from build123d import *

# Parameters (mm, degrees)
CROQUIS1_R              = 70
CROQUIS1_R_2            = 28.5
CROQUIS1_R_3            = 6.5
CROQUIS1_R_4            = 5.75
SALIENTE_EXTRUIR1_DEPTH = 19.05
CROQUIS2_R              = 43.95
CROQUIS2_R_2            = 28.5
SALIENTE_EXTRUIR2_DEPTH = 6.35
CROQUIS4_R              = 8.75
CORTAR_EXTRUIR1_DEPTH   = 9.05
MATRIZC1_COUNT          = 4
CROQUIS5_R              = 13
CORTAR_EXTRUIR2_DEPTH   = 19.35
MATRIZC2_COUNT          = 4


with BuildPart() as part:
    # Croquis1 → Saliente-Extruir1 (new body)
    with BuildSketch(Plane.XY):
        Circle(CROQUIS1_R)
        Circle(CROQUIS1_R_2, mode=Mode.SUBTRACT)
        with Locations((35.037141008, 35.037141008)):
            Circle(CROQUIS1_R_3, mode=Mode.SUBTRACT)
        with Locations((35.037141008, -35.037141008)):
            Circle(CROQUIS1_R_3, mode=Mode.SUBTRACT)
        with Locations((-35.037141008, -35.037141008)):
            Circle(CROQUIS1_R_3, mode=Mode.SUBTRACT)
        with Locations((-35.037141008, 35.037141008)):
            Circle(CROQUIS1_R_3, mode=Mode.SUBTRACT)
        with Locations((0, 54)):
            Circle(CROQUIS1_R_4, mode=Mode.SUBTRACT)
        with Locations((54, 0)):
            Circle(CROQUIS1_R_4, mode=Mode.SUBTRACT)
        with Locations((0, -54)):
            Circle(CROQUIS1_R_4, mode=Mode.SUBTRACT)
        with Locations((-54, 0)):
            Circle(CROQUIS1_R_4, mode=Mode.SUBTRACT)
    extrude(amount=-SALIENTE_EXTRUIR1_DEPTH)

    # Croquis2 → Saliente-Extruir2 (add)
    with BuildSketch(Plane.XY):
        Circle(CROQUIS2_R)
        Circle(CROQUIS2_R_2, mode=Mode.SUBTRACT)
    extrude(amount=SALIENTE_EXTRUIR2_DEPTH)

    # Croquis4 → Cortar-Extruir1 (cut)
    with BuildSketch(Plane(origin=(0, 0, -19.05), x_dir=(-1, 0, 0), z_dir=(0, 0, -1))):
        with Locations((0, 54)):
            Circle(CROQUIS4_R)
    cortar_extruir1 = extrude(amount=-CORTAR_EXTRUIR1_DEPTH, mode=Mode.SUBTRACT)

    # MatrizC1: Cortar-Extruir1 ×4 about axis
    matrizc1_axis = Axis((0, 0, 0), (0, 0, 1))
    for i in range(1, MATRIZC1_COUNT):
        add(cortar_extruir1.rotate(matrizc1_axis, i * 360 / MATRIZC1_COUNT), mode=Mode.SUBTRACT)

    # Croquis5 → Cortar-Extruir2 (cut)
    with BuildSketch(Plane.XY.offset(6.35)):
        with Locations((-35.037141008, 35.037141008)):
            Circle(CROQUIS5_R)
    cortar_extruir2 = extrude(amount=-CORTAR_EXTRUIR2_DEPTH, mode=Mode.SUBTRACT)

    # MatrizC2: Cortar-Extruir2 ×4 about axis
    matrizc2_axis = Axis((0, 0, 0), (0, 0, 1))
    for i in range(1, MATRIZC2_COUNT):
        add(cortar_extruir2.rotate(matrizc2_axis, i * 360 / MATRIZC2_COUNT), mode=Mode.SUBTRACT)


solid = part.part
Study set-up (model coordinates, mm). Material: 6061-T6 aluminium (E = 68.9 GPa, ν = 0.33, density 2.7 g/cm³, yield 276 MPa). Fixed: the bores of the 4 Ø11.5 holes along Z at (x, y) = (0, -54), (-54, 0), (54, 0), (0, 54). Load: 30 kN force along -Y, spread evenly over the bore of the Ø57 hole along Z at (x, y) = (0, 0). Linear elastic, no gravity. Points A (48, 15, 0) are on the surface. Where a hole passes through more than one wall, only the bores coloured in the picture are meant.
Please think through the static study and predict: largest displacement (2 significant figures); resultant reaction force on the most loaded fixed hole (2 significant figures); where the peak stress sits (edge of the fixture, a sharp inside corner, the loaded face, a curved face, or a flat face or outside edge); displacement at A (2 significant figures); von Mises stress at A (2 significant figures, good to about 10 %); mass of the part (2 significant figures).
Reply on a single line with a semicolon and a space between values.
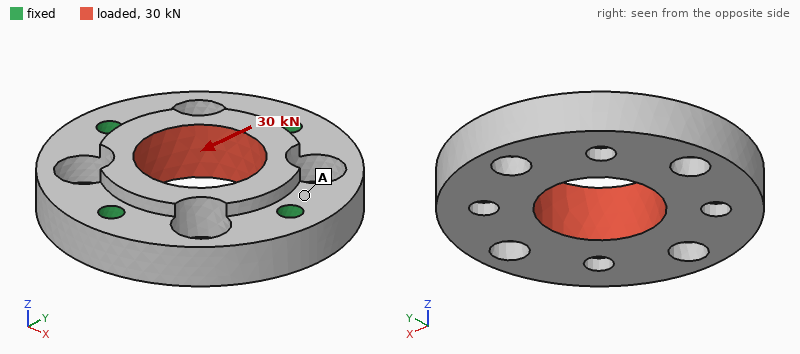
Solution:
13 µm; 8.8 kN; edge of the fixture; 3.7 µm; 9.8 MPa; 600 g
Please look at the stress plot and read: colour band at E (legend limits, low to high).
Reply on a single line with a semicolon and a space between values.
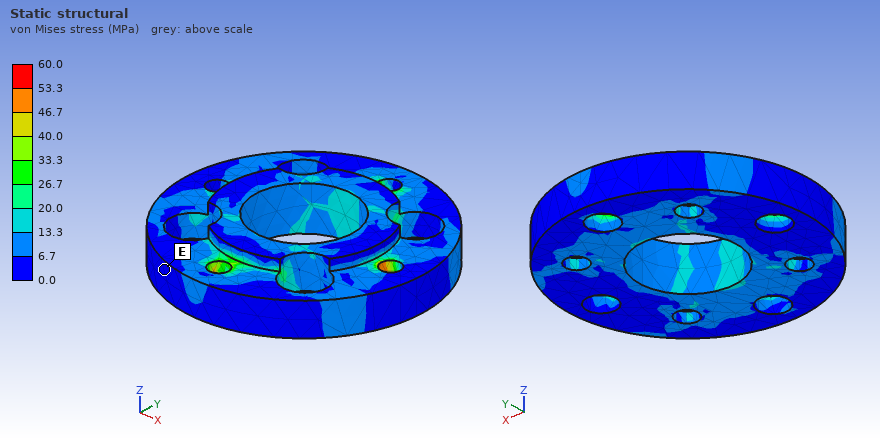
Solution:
0.0 to 6.7 MPa
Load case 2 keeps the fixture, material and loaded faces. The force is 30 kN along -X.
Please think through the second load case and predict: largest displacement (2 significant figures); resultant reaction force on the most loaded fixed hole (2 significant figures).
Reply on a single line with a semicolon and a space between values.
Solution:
13 µm; 8.7 kN
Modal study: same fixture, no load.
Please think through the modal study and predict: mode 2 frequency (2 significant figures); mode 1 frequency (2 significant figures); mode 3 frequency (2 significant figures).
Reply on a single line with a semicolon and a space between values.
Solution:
8600 Hz; 7200 Hz; 8600 Hz
